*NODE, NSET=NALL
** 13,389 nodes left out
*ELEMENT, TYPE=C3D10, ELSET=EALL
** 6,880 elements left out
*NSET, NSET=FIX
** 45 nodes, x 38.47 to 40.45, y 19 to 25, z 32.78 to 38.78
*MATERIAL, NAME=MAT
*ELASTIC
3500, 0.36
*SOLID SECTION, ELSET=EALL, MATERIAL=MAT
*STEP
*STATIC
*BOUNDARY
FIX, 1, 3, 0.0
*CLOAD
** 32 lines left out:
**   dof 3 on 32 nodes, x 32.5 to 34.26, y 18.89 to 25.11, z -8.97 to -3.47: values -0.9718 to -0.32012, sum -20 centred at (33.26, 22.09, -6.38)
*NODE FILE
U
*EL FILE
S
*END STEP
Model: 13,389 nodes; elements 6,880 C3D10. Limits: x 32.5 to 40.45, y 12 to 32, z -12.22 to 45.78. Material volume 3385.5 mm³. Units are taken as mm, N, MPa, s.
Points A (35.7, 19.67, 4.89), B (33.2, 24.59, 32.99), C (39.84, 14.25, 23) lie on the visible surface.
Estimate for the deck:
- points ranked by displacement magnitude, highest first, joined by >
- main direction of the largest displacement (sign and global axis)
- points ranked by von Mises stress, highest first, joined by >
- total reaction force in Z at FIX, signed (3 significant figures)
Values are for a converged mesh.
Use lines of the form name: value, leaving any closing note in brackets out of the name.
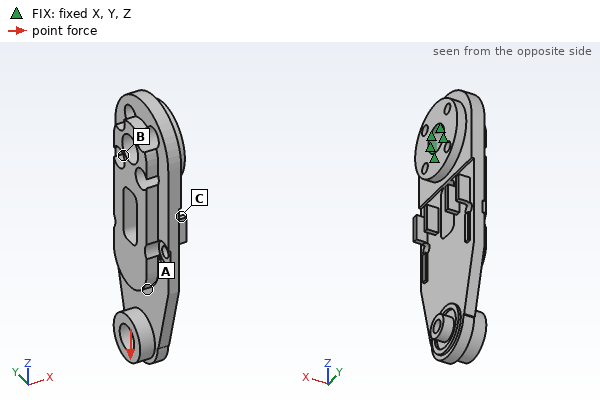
points ranked by displacement magnitude, highest first, joined by >: A > C > B
main direction of the largest displacement: +X
points ranked by von Mises stress, highest first, joined by >: A > B > C
total reaction force in Z at FIX, signed: 20.0 N
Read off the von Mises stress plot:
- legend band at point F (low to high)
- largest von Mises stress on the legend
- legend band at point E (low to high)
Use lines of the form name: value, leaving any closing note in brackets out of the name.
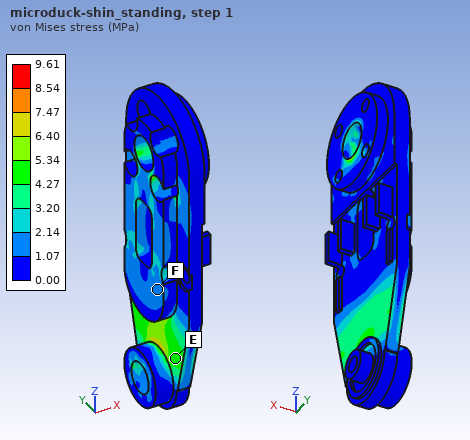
legend band at point F: 1.07 to 2.14 MPa
largest von Mises stress on the legend: 9.61 MPa
legend band at point E: 4.27 to 5.34 MPa
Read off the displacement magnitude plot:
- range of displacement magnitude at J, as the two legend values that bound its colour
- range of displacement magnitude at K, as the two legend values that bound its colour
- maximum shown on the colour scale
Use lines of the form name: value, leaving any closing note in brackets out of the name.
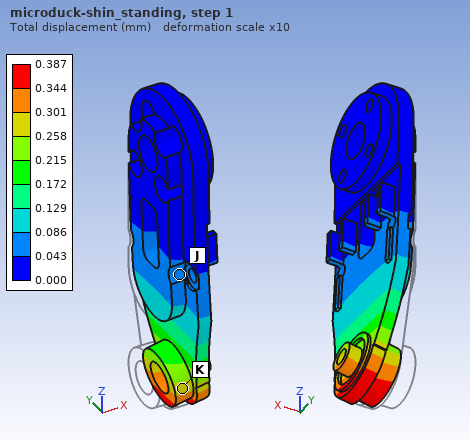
range of displacement magnitude at J, as the two legend values that bound its colour: 0.043 to 0.086 mm
range of displacement magnitude at K, as the two legend values that bound its colour: 0.258 to 0.301 mm
maximum shown on the colour scale: 0.387 mm
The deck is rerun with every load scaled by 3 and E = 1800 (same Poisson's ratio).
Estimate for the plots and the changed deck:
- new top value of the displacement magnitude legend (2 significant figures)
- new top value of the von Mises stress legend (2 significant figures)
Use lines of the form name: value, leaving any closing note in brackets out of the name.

new top value of the displacement magnitude legend: 2.3 mm
new top value of the von Mises stress legend: 29 MPa
